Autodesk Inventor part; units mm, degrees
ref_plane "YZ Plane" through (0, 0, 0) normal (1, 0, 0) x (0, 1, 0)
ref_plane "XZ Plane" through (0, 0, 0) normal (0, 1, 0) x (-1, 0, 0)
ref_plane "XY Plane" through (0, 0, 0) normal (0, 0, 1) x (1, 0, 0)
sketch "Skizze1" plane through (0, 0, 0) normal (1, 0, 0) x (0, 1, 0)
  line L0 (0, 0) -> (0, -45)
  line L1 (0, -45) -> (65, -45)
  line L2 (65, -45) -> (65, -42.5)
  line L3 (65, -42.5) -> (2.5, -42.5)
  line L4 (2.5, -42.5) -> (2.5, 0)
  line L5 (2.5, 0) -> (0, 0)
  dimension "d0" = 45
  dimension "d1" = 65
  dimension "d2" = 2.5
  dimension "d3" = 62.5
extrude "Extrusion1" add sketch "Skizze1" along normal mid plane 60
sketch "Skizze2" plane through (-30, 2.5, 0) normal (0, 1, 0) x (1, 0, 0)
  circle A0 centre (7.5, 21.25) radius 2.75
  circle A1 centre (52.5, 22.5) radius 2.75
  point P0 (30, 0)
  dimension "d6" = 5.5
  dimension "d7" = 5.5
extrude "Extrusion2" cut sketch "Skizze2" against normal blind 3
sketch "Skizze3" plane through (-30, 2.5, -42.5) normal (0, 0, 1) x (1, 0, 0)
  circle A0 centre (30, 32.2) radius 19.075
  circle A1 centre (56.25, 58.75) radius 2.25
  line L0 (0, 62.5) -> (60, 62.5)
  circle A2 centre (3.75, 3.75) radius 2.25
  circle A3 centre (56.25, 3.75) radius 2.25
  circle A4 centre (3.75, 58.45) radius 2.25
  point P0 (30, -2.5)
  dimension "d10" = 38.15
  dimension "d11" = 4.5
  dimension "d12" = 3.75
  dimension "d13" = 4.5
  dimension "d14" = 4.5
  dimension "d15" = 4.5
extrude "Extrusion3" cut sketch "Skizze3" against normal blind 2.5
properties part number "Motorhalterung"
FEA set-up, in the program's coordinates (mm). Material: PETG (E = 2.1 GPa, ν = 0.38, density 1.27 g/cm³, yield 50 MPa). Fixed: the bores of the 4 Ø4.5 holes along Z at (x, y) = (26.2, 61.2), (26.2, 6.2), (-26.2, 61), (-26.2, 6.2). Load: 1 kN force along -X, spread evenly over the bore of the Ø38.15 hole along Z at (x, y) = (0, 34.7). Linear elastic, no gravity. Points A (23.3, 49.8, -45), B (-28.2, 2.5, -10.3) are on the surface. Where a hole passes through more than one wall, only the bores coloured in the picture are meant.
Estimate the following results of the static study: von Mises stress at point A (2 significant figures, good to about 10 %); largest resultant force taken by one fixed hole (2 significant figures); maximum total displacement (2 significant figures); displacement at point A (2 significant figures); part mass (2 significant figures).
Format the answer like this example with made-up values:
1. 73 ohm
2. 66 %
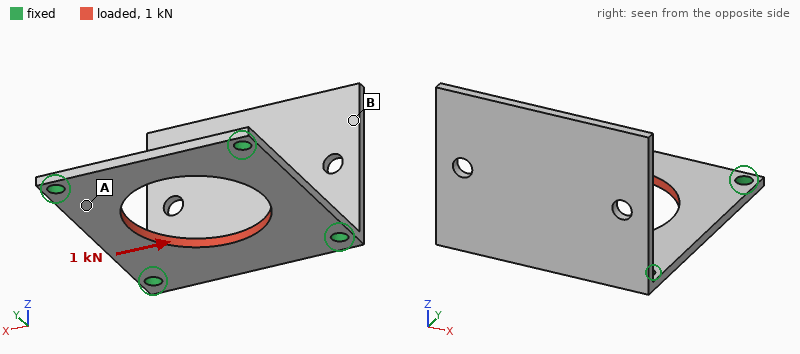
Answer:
1. 5.4 MPa
2. 280 N
3. 0.21 mm
4. 0.10 mm
5. 16 g
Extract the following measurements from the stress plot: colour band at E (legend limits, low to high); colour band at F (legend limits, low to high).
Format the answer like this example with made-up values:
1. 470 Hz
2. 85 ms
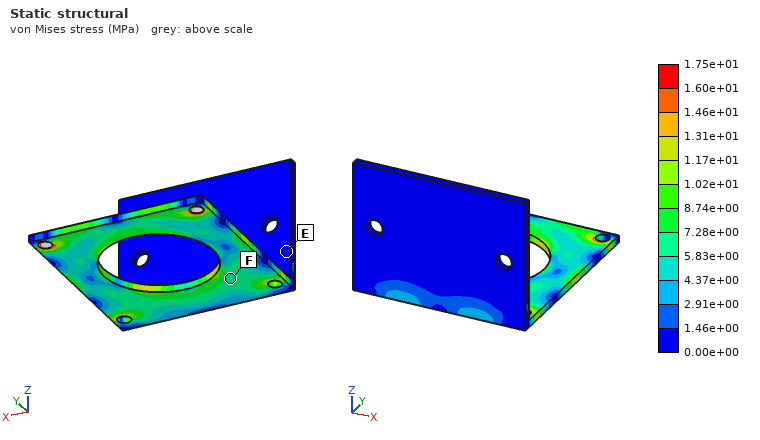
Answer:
1. 0.00e+00 to 1.46e+00 MPa
2. 5.83e+00 to 7.28e+00 MPa
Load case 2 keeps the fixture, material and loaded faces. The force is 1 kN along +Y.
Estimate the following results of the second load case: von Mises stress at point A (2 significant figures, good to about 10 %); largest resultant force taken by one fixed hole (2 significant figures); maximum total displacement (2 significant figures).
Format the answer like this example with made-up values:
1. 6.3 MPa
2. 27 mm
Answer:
1. 5.1 MPa
2. 260 N
3. 0.23 mm
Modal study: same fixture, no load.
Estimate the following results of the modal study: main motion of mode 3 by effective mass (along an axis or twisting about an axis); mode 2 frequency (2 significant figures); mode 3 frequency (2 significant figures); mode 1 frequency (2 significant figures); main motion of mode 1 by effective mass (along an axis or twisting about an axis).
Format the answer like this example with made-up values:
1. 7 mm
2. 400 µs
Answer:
1. along Z
2. 490 Hz
3. 1200 Hz
4. 220 Hz
5. along Y
